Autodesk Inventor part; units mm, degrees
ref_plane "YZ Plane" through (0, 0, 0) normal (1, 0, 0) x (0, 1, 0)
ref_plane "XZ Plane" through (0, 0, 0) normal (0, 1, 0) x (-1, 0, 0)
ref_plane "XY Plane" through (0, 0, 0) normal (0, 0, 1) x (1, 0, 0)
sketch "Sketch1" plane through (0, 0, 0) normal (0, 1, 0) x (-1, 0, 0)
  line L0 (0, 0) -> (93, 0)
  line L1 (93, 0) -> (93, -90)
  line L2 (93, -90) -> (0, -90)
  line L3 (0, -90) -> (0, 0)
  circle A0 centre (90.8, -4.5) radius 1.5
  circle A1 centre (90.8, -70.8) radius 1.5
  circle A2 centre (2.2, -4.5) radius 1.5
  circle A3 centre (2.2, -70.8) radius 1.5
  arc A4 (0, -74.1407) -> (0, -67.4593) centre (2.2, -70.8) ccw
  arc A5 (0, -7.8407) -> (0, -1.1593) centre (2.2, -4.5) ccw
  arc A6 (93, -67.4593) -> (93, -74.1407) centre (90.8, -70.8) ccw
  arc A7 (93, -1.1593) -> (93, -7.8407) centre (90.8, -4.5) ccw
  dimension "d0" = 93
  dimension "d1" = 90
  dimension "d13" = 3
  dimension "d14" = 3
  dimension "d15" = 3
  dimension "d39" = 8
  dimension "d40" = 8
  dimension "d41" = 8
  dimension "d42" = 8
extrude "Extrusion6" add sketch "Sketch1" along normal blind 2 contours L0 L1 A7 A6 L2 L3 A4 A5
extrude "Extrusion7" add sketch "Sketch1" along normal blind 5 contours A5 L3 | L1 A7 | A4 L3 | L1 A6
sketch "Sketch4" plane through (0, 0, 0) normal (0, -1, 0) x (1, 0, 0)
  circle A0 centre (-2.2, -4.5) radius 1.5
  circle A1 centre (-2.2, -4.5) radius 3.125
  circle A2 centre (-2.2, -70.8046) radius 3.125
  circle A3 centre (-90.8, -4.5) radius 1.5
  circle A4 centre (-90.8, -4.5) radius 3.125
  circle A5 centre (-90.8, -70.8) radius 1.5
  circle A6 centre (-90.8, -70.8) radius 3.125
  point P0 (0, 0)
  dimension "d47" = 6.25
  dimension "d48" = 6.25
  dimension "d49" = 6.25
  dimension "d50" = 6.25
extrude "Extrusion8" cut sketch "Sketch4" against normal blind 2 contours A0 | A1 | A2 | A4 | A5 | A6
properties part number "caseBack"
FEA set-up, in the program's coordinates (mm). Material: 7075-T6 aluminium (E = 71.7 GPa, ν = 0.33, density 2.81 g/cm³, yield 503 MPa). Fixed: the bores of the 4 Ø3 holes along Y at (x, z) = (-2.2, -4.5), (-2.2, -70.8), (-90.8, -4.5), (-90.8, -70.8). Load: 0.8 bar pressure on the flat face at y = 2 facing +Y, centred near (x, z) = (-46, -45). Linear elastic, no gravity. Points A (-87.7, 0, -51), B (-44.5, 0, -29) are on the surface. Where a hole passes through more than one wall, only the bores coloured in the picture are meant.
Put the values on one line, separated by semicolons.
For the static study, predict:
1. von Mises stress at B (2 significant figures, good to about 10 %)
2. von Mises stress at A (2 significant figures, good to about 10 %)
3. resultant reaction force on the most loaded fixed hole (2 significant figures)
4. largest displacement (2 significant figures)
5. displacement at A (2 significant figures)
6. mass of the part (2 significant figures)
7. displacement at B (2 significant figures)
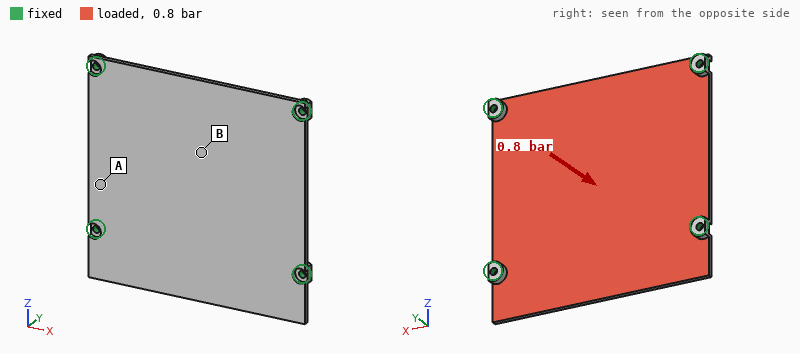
46 MPa; 20 MPa; 520 N; 0.45 mm; 0.10 mm; 48 g; 0.45 mm
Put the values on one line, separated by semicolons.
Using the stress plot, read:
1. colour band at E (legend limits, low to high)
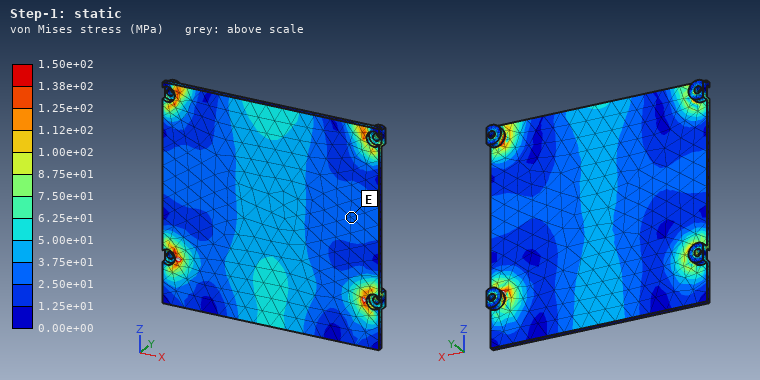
2.50e+01 to 3.75e+01 MPa
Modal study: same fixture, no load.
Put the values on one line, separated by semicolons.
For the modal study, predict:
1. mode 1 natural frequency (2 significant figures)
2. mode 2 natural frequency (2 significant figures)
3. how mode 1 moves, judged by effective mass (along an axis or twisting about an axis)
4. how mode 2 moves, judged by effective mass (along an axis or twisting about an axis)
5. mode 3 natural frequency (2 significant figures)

1100 Hz; 1400 Hz; along Y; twisting about X; 2100 Hz
